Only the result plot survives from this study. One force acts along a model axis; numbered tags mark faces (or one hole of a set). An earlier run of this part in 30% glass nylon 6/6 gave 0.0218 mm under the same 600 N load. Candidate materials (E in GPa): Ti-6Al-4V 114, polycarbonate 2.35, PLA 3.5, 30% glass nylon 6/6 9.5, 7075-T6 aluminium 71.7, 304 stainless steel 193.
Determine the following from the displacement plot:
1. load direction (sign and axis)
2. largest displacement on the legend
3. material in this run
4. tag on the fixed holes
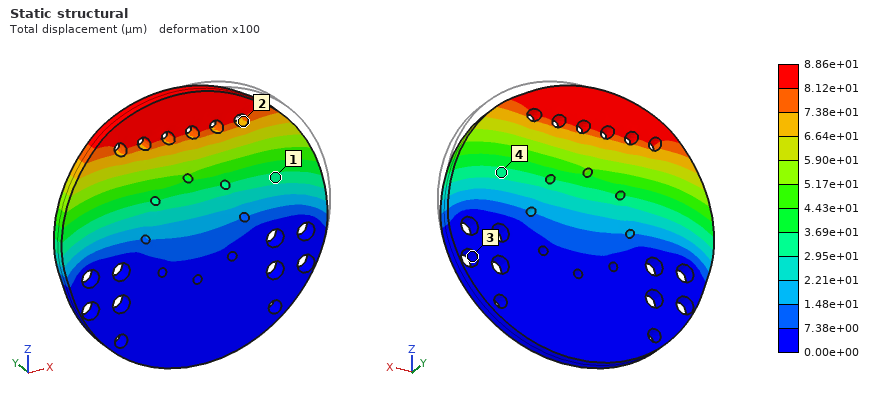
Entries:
-X
8.86e+01 µm
polycarbonate
3
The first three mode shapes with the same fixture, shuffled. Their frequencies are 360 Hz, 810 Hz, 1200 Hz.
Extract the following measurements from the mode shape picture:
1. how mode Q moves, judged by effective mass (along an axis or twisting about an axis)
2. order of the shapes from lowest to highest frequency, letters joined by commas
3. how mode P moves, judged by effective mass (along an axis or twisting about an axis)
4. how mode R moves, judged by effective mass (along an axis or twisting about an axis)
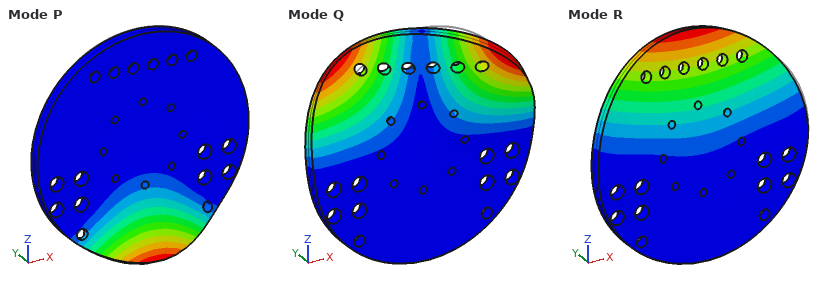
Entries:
twisting about Z
R, Q, P
along Y
along Y
